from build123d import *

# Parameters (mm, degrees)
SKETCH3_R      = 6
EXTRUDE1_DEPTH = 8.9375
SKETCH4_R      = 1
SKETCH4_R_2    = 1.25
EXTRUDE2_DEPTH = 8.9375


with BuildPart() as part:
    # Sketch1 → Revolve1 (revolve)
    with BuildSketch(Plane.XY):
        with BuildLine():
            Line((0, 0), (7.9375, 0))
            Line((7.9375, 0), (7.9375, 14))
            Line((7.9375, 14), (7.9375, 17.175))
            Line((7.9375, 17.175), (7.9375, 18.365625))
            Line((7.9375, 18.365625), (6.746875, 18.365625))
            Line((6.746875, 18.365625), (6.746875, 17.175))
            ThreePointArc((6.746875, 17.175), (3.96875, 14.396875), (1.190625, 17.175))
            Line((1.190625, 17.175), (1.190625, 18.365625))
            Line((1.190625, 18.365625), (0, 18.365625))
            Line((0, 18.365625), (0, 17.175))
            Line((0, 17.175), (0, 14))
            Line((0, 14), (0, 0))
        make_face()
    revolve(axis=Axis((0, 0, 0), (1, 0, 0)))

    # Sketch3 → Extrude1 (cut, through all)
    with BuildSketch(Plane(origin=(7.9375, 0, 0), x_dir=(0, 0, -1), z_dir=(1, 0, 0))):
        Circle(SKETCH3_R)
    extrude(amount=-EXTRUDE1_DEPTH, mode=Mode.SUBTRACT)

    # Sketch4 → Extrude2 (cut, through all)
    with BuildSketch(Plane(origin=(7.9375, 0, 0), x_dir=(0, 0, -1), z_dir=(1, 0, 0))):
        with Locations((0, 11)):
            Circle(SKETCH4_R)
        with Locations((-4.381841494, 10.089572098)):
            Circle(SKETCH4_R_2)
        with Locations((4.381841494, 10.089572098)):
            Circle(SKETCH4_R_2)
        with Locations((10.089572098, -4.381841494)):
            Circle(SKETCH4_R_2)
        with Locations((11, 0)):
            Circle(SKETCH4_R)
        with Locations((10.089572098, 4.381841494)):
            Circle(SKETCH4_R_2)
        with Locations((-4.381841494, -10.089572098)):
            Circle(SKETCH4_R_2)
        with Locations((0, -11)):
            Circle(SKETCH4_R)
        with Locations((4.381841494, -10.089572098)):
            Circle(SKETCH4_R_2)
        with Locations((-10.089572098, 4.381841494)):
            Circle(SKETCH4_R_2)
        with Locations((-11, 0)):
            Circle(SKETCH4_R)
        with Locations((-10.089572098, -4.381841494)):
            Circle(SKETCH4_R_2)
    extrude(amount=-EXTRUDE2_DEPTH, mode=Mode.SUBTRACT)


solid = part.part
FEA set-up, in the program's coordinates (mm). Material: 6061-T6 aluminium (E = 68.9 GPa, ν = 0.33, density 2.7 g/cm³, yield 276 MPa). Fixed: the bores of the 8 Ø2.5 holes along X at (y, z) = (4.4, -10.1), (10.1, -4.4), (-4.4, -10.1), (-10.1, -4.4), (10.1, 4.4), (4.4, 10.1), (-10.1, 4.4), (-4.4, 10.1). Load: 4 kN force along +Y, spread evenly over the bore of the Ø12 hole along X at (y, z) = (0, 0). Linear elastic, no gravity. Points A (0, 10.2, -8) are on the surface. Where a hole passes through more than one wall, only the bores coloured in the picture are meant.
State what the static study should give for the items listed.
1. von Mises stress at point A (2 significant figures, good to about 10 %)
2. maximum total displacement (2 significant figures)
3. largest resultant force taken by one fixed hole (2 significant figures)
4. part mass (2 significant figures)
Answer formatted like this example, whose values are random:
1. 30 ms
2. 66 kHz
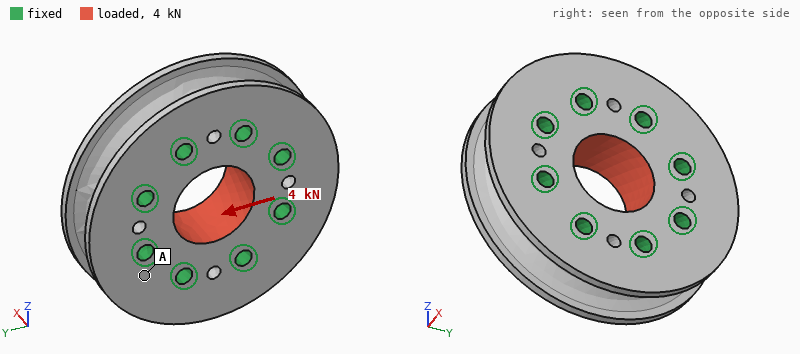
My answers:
1. 3.2 MPa
2. 1.2 µm
3. 710 N
4. 14 g
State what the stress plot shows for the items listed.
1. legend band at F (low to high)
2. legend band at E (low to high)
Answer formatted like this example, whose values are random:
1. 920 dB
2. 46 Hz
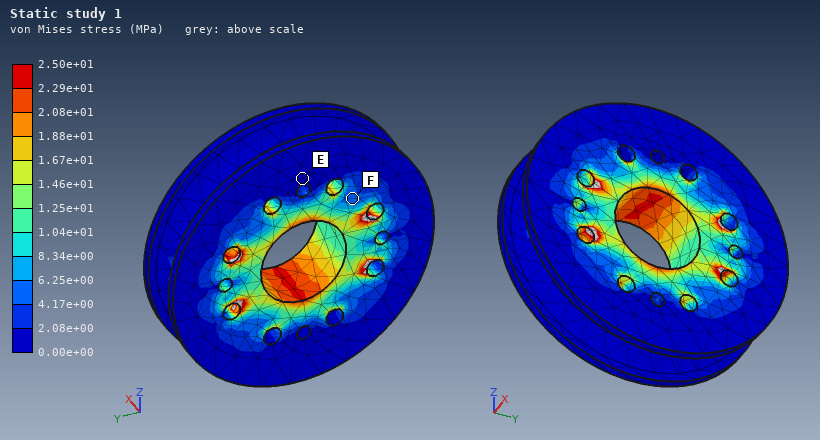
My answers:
1. 4.17e+00 to 6.25e+00 MPa
2. 0.00e+00 to 2.08e+00 MPa
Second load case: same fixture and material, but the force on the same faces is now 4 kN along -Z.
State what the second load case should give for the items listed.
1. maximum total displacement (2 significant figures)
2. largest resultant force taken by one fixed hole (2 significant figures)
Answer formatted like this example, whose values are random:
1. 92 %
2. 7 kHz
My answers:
1. 1.3 µm
2. 710 N
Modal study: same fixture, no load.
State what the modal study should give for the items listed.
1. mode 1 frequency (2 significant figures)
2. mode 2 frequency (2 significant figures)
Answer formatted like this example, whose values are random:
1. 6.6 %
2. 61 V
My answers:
1. 71 kHz
2. 71 kHz
